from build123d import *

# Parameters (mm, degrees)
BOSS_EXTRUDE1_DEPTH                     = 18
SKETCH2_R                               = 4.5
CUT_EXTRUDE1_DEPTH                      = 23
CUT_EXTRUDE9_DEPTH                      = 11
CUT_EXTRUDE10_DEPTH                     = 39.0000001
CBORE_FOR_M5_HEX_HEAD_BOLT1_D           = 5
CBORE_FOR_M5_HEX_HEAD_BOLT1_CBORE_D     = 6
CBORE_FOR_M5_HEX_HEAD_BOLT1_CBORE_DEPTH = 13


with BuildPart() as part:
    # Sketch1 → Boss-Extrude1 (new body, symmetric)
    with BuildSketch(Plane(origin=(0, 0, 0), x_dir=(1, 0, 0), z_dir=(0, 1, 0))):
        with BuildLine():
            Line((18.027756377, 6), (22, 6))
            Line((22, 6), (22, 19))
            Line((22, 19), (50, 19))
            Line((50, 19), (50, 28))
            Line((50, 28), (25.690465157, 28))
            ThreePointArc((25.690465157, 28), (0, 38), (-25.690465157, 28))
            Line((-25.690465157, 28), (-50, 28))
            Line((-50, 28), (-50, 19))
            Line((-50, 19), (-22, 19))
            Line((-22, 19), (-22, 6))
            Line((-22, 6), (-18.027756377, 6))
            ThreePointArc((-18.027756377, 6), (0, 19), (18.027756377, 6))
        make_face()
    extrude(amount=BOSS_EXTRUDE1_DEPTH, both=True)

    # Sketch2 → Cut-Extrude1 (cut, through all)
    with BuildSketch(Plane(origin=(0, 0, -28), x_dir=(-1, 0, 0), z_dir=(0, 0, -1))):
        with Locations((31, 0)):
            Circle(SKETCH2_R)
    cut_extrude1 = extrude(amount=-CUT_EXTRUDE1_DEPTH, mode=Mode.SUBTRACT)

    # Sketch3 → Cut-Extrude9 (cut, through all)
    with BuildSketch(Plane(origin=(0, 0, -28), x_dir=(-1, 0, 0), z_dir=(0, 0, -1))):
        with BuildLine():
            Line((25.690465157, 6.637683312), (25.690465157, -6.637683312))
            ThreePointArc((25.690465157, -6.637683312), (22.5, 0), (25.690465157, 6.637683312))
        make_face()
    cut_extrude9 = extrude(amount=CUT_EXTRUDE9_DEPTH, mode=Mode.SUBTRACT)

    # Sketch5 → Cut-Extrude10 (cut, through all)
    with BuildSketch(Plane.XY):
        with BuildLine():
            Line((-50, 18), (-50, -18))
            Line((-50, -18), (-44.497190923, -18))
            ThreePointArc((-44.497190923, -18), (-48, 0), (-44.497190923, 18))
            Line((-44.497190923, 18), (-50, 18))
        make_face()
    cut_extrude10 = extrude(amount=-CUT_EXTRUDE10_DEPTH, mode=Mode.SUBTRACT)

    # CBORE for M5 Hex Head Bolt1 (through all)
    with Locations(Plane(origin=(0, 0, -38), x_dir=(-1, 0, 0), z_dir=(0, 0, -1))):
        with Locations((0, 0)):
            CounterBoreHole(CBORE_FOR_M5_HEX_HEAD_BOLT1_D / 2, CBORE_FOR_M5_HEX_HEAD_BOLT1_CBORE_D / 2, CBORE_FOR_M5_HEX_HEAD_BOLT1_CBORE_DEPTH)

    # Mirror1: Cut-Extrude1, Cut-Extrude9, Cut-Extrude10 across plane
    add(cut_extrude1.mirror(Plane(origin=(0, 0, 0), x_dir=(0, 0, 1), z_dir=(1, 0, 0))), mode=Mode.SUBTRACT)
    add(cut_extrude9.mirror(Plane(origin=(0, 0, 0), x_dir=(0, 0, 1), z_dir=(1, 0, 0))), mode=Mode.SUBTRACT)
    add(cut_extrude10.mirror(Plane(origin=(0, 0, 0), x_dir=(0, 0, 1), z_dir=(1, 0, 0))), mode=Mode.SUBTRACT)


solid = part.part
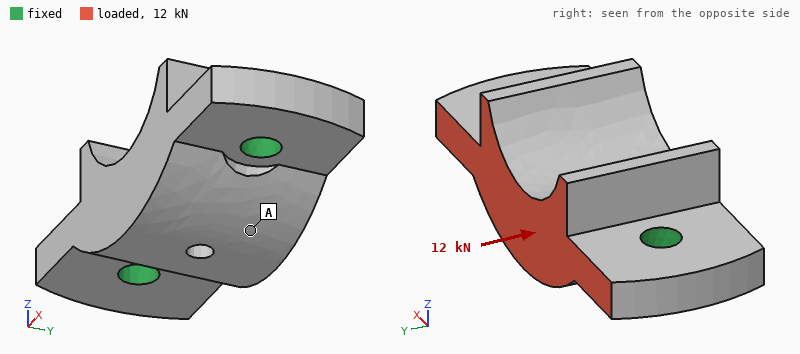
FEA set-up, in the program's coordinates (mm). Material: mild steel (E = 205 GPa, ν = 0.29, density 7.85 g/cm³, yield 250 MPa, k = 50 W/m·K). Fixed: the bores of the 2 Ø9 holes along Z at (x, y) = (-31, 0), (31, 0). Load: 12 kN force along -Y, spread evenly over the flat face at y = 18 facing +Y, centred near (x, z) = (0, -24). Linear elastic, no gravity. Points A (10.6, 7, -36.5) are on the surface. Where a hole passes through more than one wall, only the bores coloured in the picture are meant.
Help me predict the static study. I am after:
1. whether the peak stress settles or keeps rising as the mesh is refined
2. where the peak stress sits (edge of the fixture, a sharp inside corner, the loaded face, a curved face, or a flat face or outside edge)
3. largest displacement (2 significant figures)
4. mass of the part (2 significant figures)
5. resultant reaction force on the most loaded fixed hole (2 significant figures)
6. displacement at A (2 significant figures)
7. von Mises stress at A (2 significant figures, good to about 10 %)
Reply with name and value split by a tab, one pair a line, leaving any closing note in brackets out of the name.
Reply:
whether the peak stress settles or keeps rising as the mesh is refined	keeps rising
where the peak stress sits	edge of the fixture
largest displacement	6.0 µm
mass of the part	390 g
resultant reaction force on the most loaded fixed hole	6.0 kN
displacement at A	4.8 µm
von Mises stress at A	10 MPa
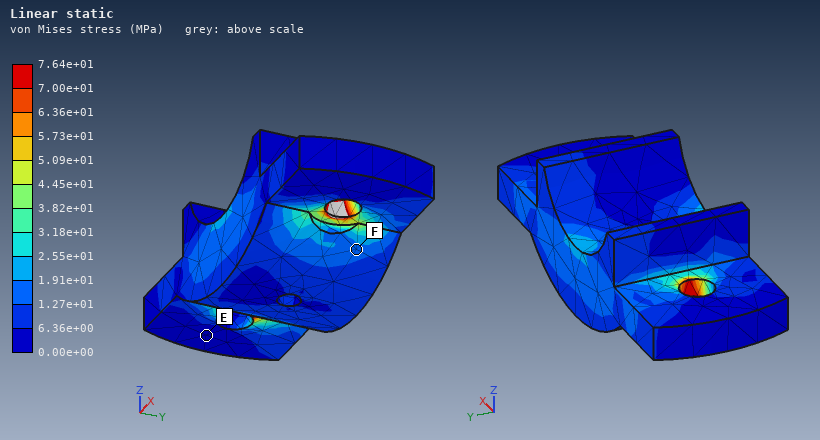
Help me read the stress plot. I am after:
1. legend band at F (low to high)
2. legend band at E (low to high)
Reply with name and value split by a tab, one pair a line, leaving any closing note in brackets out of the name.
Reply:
legend band at F	1.27e+01 to 1.91e+01 MPa
legend band at E	0.00e+00 to 6.36e+00 MPa
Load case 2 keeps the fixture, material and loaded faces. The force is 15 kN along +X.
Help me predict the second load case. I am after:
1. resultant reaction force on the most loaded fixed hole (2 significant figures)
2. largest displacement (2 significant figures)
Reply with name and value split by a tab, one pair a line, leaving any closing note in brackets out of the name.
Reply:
resultant reaction force on the most loaded fixed hole	8.5 kN
largest displacement	8.4 µm
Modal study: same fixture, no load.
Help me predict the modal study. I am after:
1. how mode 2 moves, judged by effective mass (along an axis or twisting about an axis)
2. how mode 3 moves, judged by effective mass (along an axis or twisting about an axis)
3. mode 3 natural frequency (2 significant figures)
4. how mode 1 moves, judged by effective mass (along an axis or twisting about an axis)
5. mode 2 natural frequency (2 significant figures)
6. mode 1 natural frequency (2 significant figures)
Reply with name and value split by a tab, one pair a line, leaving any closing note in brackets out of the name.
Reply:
how mode 2 moves, judged by effective mass	along Z
how mode 3 moves, judged by effective mass	along Y
mode 3 natural frequency	15 kHz
how mode 1 moves, judged by effective mass	twisting about X
mode 2 natural frequency	12 kHz
mode 1 natural frequency	9100 Hz
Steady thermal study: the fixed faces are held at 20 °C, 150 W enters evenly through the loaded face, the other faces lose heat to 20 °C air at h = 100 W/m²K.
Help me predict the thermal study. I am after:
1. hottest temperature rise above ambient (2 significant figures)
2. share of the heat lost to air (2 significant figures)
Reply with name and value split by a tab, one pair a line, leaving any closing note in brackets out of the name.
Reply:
hottest temperature rise above ambient	72 K
share of the heat lost to air	20 %
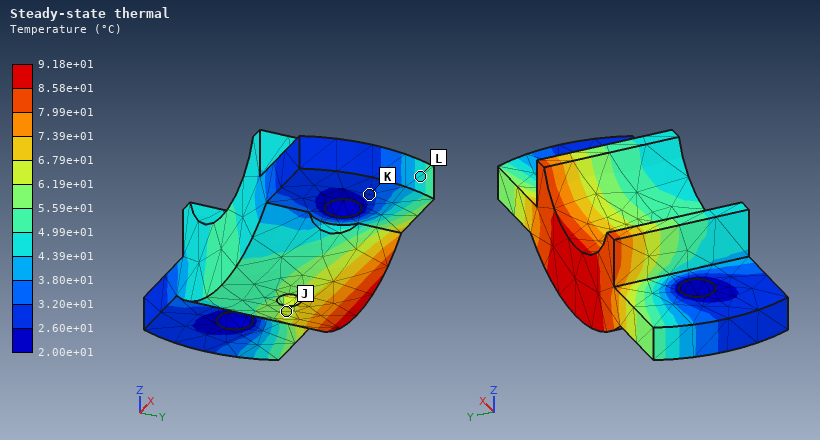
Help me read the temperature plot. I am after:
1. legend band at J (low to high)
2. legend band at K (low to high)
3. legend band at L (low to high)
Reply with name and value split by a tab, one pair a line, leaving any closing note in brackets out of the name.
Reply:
legend band at J	6.19e+01 to 6.79e+01 °C
legend band at K	2.60e+01 to 3.20e+01 °C
legend band at L	4.39e+01 to 4.99e+01 °C
